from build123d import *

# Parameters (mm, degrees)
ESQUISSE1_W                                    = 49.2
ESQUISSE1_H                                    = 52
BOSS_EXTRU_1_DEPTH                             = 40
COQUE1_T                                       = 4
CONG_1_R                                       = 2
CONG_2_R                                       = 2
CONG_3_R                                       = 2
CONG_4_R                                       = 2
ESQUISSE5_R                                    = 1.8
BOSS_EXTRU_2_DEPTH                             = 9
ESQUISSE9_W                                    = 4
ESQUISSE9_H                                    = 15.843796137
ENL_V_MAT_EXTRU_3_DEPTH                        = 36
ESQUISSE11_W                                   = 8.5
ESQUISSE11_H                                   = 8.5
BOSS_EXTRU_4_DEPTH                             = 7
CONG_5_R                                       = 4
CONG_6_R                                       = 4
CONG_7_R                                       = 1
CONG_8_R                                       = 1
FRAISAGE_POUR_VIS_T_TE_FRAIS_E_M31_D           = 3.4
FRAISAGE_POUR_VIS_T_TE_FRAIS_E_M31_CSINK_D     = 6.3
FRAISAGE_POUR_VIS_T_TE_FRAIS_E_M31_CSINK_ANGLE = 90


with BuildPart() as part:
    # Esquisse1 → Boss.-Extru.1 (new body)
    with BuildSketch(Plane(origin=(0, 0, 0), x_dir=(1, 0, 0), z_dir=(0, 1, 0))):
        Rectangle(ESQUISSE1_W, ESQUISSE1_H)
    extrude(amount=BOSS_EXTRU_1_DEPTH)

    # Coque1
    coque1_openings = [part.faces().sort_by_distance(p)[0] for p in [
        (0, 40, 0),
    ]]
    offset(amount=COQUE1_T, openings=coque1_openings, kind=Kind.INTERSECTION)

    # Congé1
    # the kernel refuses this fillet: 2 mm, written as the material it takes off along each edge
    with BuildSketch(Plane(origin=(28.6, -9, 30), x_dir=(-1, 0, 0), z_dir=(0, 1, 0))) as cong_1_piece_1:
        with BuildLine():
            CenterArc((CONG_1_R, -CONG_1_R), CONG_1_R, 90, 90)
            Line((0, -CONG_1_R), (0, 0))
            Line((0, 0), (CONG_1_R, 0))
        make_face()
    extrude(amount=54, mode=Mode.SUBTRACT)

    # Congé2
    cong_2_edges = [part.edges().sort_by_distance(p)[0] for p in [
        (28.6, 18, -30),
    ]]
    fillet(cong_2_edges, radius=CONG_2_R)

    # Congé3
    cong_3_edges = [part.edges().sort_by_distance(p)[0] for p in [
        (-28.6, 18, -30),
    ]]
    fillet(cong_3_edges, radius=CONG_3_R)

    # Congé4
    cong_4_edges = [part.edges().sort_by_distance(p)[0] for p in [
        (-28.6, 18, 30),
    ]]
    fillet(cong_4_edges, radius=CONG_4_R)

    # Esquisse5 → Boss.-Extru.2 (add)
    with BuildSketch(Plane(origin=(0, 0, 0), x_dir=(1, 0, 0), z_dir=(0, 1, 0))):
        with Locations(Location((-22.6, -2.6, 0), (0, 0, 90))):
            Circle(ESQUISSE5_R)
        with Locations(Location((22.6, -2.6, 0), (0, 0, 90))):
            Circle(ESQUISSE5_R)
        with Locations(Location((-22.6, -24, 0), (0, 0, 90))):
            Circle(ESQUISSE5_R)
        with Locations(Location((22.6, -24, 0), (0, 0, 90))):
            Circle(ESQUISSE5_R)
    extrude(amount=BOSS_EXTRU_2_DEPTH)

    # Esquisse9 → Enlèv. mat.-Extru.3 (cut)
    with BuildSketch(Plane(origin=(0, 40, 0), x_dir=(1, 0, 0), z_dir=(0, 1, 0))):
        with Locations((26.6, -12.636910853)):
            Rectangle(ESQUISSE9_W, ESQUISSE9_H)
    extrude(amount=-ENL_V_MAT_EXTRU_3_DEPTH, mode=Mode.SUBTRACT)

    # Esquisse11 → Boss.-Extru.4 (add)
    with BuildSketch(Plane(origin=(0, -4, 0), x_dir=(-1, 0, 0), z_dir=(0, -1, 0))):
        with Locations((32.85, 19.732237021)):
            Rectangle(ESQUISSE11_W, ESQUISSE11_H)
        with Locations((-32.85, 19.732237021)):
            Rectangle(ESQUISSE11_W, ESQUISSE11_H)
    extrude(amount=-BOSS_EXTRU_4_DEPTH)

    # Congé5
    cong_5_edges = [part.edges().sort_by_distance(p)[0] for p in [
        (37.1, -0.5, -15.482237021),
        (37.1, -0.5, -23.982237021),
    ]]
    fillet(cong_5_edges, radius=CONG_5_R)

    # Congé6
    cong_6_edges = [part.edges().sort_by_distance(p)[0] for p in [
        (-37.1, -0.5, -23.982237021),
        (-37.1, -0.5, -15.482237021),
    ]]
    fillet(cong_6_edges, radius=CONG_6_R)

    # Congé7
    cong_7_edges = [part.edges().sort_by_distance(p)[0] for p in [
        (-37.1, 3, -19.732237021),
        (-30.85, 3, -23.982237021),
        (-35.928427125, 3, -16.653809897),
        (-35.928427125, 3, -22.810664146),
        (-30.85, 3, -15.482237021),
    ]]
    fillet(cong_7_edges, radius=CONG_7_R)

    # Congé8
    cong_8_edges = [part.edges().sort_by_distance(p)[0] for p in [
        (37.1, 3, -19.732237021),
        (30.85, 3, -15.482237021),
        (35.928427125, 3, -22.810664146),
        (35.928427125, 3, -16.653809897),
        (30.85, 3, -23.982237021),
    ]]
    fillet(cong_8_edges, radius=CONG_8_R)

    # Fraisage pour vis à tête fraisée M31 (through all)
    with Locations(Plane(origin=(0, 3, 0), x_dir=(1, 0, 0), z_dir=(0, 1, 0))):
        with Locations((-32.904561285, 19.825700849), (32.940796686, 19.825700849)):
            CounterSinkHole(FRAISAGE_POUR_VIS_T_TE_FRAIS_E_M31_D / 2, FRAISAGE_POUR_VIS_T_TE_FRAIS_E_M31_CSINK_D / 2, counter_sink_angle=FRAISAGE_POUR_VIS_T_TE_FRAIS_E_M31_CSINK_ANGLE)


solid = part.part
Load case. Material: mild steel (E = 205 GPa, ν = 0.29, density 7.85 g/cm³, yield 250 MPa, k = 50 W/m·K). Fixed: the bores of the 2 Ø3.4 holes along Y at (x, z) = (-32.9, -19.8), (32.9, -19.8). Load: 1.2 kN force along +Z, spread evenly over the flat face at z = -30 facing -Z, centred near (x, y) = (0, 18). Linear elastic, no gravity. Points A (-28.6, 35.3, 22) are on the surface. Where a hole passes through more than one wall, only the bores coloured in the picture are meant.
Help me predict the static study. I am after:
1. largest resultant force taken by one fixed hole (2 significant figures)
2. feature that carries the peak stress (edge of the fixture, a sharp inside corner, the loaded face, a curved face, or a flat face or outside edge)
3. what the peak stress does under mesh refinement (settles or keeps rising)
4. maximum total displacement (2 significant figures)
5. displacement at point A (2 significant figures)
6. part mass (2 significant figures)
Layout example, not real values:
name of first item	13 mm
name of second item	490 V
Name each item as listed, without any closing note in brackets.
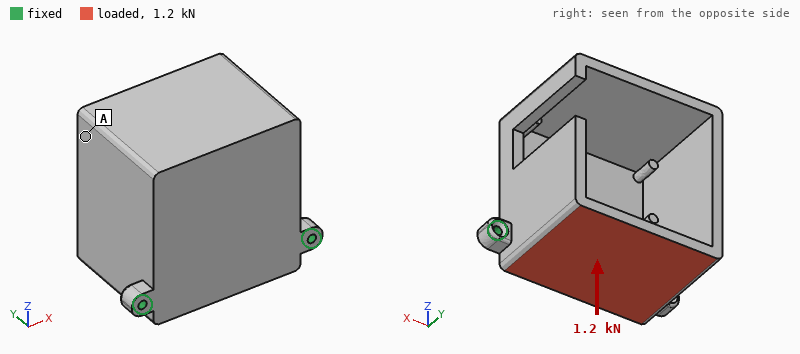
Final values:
largest resultant force taken by one fixed hole	600 N
feature that carries the peak stress	edge of the fixture
what the peak stress does under mesh refinement	keeps rising
maximum total displacement	0.12 mm
displacement at point A	0.10 mm
part mass	370 g
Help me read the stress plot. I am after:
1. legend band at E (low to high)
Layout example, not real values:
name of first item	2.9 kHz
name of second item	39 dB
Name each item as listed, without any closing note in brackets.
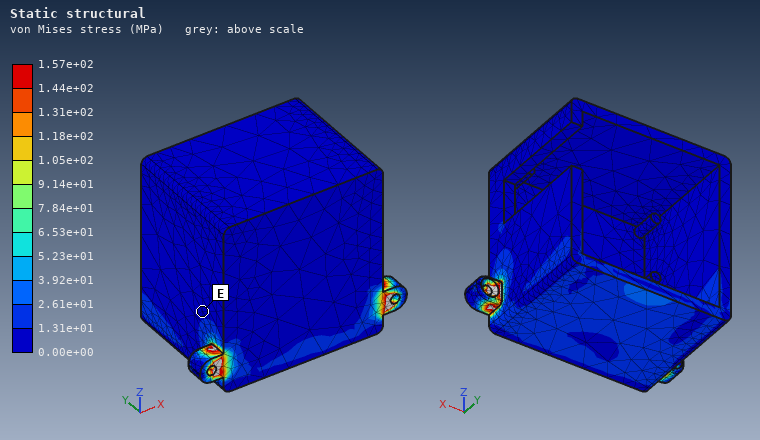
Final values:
legend band at E	0.00e+00 to 1.31e+01 MPa
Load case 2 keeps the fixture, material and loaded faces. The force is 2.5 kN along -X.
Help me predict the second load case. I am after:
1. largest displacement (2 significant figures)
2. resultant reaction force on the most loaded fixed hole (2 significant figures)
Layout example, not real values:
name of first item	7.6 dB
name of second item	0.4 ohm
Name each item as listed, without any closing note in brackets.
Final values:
largest displacement	13 µm
resultant reaction force on the most loaded fixed hole	1.5 kN
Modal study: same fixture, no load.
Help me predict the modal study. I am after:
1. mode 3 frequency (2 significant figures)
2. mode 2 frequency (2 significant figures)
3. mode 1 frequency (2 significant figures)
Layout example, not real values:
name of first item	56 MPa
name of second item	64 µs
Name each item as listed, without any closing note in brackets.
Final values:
mode 3 frequency	2600 Hz
mode 2 frequency	1700 Hz
mode 1 frequency	800 Hz
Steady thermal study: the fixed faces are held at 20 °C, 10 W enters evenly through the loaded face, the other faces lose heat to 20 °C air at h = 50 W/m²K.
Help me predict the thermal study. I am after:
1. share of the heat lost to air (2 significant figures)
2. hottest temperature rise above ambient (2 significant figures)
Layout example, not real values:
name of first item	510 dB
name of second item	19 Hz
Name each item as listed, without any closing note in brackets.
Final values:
share of the heat lost to air	56 %
hottest temperature rise above ambient	15 K
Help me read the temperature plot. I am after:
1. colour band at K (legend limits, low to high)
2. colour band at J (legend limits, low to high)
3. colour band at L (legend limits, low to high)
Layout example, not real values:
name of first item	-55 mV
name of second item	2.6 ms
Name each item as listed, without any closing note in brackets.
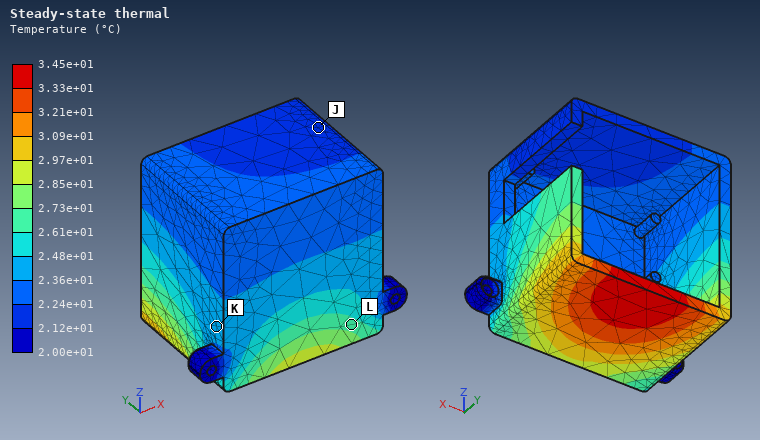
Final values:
colour band at K	2.36e+01 to 2.48e+01 °C
colour band at J	2.12e+01 to 2.24e+01 °C
colour band at L	2.61e+01 to 2.73e+01 °C
